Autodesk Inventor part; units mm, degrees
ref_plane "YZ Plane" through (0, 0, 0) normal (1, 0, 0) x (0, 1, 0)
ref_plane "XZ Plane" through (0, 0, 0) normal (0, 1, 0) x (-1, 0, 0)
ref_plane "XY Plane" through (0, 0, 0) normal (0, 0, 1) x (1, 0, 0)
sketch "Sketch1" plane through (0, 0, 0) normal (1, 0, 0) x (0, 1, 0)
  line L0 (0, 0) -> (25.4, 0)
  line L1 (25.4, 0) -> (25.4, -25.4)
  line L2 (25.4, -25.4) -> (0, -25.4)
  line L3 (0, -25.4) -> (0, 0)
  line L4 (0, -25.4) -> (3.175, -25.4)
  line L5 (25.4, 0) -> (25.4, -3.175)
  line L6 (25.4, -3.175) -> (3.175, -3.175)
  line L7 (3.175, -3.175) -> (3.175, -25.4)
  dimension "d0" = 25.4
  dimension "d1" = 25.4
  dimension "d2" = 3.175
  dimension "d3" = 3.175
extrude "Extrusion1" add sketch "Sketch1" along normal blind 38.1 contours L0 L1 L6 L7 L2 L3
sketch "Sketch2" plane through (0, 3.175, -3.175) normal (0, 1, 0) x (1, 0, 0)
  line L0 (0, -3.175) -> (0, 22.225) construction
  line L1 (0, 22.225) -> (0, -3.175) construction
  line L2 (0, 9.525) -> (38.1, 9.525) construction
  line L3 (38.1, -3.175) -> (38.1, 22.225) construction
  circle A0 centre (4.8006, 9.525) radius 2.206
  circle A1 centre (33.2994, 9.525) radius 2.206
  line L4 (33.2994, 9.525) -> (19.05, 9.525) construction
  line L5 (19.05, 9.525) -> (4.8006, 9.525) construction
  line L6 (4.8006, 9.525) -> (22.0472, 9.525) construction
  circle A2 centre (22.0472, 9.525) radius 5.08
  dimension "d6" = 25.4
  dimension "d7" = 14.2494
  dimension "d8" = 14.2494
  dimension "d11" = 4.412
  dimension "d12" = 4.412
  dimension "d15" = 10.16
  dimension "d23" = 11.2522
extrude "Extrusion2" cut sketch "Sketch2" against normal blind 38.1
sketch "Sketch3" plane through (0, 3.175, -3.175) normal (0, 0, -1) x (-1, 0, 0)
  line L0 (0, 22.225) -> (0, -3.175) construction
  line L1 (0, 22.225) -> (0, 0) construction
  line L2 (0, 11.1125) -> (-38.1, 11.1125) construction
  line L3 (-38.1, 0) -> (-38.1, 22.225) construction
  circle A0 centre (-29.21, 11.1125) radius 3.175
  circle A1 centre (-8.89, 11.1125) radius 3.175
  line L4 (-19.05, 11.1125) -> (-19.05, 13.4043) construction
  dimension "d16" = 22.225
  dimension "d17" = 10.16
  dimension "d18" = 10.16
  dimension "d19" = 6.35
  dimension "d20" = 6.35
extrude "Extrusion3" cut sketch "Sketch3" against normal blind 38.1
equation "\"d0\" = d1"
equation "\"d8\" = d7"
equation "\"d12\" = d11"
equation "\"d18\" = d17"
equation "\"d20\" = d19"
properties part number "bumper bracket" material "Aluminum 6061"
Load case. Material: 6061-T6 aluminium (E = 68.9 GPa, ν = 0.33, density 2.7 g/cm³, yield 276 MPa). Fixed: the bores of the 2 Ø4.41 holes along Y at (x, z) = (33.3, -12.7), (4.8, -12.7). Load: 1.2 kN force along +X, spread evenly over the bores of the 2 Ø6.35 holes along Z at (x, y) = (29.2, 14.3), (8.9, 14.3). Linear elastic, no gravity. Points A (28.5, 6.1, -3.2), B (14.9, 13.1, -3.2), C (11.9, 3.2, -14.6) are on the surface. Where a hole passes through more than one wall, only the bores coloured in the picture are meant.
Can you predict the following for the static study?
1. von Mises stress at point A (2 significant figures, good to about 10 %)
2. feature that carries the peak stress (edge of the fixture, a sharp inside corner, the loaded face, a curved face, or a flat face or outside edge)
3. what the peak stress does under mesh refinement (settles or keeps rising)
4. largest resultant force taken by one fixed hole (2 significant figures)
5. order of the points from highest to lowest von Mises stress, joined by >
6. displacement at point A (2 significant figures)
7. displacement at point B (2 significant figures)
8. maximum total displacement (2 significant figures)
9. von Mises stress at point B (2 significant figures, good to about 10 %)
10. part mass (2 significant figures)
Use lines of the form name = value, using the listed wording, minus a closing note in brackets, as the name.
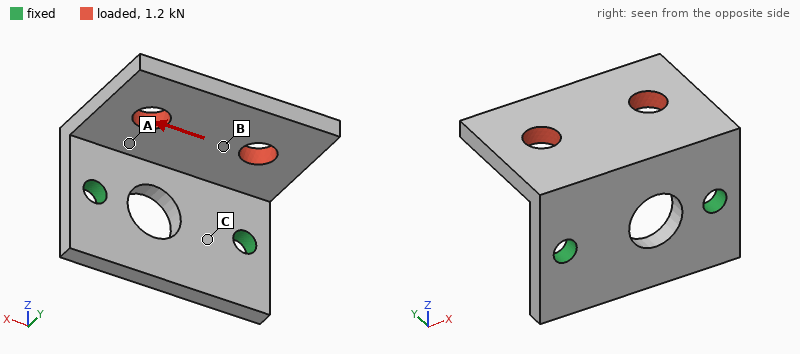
von Mises stress at point A = 62 MPa
feature that carries the peak stress = edge of the fixture
what the peak stress does under mesh refinement = keeps rising
largest resultant force taken by one fixed hole = 930 N
order of the points from highest to lowest von Mises stress, joined by > = A > B > C
displacement at point A = 0.036 mm
displacement at point B = 0.051 mm
maximum total displacement = 0.12 mm
von Mises stress at point B = 38 MPa
part mass = 14 g
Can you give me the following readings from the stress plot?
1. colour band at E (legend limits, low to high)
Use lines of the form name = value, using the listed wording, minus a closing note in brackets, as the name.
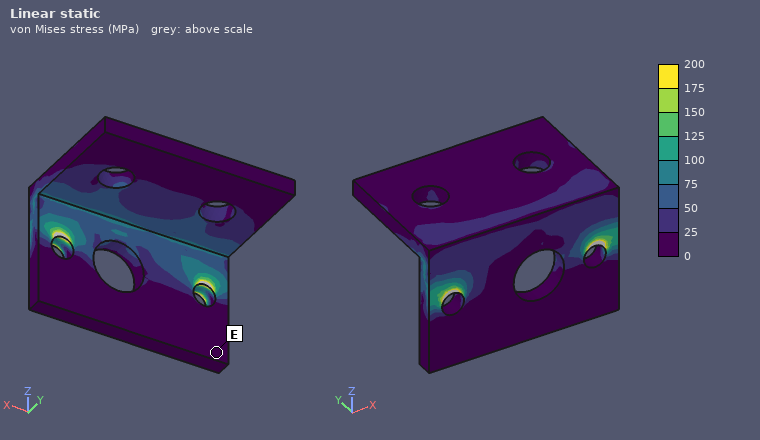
colour band at E = 0 to 25 MPa
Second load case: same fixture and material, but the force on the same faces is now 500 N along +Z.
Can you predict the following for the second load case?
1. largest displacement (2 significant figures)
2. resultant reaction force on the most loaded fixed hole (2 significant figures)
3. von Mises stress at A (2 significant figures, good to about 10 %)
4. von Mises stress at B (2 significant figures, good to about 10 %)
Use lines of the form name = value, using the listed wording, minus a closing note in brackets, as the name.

largest displacement = 0.35 mm
resultant reaction force on the most loaded fixed hole = 260 N
von Mises stress at A = 57 MPa
von Mises stress at B = 21 MPa
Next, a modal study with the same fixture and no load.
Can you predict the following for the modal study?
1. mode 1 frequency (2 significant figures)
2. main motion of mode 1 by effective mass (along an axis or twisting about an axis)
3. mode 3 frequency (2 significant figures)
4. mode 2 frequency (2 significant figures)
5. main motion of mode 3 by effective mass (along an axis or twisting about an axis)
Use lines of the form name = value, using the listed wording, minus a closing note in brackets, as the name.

mode 1 frequency = 2700 Hz
main motion of mode 1 by effective mass = along Z
mode 3 frequency = 8700 Hz
mode 2 frequency = 5700 Hz
main motion of mode 3 by effective mass = along X
